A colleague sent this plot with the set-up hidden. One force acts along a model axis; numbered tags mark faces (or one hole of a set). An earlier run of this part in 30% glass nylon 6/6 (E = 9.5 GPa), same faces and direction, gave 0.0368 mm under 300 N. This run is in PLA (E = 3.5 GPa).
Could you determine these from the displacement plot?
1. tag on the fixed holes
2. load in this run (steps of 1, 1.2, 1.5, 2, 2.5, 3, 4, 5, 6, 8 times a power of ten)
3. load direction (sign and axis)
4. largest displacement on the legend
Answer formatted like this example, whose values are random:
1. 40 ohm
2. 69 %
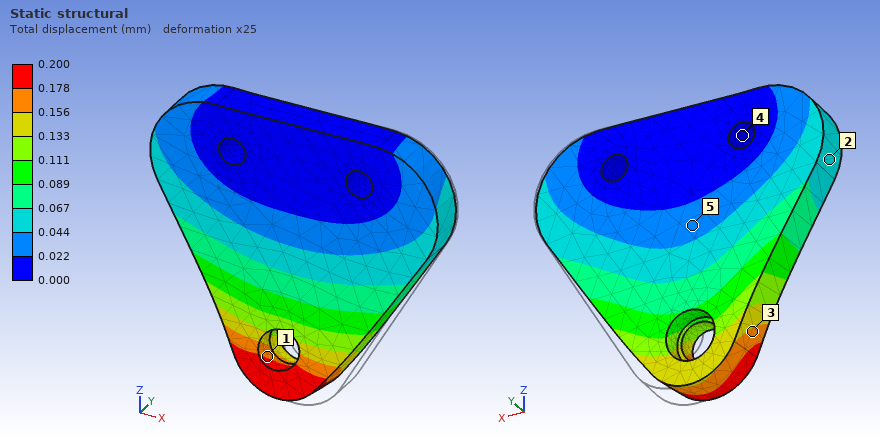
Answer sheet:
1. 4
2. 600 N
3. -X
4. 0.200 mm
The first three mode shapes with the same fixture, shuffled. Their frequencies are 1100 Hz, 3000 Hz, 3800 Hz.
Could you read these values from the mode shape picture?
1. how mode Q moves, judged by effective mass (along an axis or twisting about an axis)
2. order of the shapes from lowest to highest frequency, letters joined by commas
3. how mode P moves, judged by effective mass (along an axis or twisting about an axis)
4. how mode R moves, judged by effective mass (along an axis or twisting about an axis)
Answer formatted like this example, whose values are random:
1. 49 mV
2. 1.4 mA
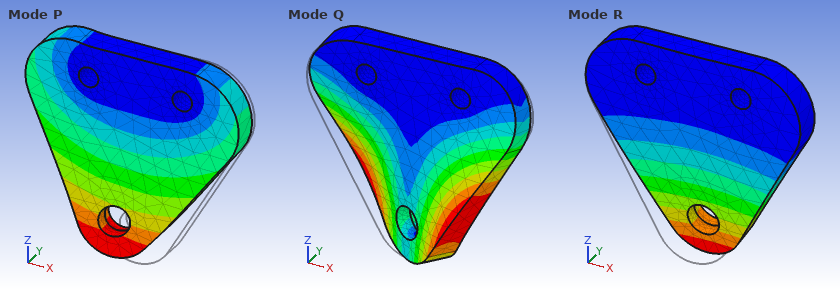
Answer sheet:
1. twisting about Z
2. R, Q, P
3. along X
4. along Y
